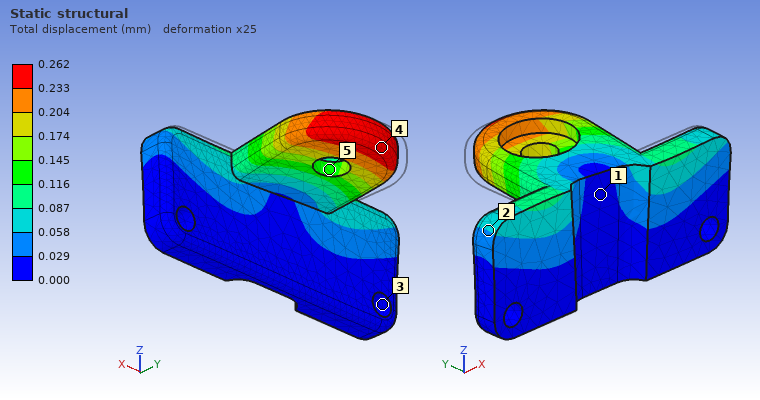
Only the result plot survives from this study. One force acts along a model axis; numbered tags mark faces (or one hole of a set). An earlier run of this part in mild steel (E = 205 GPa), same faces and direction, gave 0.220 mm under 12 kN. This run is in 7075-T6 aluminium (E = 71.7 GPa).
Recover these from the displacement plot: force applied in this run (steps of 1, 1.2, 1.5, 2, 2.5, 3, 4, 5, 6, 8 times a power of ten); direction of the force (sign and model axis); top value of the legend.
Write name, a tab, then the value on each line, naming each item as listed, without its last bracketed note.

force applied in this run	5 kN
direction of the force	+X
top value of the legend	0.262 mm
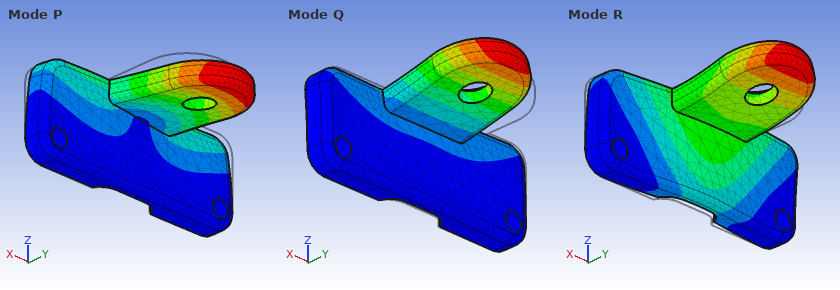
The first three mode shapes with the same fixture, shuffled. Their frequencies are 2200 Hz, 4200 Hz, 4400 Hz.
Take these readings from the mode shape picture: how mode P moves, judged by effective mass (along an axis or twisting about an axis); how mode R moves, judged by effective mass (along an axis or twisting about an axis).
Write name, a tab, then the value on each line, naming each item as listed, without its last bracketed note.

how mode P moves, judged by effective mass	along X
how mode R moves, judged by effective mass	along Y
